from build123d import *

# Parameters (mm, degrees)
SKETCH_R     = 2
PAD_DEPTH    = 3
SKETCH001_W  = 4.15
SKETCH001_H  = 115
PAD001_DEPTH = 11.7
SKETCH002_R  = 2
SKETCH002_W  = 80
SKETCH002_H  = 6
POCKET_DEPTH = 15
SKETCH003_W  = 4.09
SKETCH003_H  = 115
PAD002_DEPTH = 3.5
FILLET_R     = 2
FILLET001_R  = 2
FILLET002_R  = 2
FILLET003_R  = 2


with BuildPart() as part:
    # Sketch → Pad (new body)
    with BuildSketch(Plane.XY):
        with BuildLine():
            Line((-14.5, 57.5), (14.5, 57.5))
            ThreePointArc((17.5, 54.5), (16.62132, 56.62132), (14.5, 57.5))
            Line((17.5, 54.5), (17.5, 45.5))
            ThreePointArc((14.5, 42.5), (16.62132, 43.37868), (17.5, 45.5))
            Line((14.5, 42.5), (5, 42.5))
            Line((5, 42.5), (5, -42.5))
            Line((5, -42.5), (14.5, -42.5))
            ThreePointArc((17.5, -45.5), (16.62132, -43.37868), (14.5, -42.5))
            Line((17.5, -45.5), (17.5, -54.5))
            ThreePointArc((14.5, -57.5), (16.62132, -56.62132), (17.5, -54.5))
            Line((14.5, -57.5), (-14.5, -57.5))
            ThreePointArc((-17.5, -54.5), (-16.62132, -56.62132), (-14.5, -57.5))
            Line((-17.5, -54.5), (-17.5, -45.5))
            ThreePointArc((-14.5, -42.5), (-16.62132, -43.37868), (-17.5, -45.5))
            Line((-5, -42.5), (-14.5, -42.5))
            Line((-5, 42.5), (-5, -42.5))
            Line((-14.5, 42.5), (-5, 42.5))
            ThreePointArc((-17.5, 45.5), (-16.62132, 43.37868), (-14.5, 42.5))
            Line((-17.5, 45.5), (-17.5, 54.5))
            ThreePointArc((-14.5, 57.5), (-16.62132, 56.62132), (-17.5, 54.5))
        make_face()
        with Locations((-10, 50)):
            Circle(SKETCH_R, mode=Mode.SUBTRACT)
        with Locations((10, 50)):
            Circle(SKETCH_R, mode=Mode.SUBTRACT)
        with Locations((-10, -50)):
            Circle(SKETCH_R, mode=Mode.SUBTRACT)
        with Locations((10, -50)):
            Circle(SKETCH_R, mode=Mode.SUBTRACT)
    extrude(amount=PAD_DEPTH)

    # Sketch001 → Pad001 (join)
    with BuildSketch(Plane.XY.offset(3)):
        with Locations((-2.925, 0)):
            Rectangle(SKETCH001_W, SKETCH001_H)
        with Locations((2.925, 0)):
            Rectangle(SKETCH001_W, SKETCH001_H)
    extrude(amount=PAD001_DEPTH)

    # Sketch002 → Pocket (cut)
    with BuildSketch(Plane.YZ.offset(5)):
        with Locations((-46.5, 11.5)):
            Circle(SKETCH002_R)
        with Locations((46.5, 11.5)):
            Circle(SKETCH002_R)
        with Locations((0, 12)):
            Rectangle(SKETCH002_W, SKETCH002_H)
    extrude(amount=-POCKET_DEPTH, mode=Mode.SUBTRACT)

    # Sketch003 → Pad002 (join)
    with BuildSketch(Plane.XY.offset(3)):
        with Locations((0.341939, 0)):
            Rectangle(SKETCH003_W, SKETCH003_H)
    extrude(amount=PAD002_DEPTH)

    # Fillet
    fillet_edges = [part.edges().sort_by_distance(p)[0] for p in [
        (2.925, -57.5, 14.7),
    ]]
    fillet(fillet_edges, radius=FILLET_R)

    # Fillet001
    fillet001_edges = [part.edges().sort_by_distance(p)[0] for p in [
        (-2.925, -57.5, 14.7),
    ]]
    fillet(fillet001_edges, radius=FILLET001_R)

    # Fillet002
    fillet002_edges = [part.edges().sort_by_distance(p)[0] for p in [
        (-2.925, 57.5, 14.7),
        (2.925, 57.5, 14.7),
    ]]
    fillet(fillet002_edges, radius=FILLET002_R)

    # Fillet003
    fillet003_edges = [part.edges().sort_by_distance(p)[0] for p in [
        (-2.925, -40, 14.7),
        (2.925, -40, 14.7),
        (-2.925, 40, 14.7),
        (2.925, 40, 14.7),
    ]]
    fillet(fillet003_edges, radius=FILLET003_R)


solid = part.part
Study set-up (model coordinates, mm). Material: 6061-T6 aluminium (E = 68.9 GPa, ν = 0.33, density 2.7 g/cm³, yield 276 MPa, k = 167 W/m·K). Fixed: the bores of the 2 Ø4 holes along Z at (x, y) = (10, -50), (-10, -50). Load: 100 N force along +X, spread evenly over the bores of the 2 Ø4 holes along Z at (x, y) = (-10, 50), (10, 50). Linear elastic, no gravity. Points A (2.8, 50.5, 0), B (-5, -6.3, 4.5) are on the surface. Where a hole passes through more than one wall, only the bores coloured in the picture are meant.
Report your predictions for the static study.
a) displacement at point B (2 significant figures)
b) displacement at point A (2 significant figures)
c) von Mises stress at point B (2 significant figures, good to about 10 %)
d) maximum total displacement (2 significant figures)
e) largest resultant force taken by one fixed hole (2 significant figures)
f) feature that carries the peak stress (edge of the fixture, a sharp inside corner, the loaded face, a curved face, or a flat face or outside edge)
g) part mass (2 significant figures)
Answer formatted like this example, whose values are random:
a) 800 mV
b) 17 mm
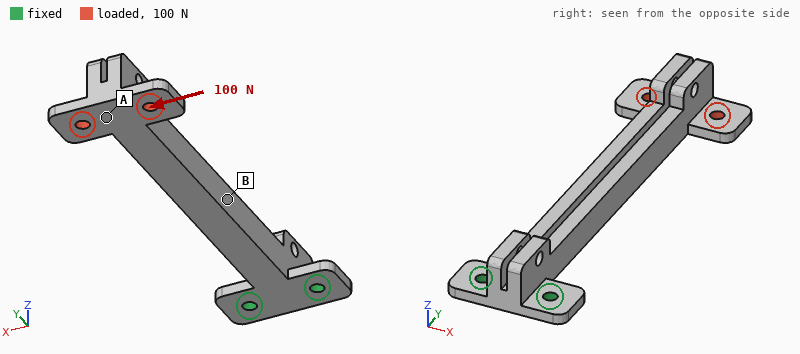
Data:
a) 0.15 mm
b) 0.63 mm
c) 38 MPa
d) 0.70 mm
e) 500 N
f) a flat face or outside edge
g) 36 g
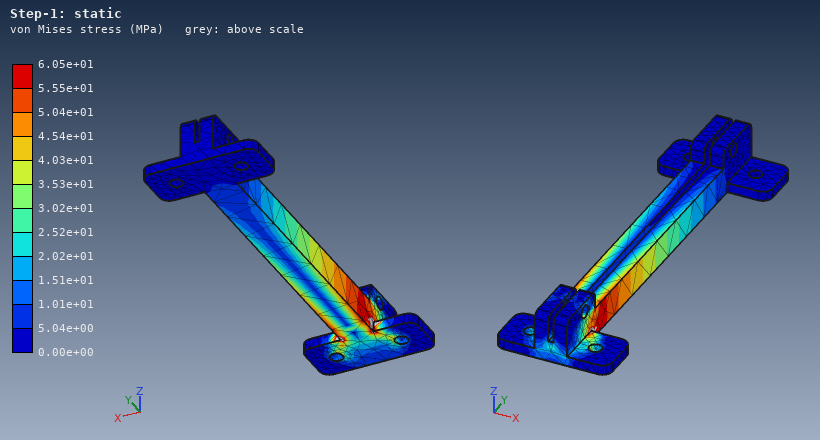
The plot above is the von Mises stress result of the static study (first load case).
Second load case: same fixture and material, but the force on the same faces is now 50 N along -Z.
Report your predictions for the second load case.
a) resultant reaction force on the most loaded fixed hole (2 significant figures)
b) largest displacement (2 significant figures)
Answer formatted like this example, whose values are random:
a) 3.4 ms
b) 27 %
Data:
a) 81 N
b) 0.72 mm
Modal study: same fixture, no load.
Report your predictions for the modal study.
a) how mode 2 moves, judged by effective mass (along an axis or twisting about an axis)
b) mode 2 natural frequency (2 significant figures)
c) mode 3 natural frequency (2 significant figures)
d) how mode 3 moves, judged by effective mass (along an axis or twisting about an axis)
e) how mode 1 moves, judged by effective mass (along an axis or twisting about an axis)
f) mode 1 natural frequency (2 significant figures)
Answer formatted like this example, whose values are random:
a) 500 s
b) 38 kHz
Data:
a) along X
b) 580 Hz
c) 2800 Hz
d) twisting about Y
e) along Z
f) 390 Hz
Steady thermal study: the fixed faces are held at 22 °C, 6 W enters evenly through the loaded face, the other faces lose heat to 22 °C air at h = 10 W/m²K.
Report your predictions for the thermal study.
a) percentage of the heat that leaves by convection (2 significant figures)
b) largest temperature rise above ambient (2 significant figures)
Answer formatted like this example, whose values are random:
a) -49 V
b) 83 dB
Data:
a) 23 %
b) 37 K
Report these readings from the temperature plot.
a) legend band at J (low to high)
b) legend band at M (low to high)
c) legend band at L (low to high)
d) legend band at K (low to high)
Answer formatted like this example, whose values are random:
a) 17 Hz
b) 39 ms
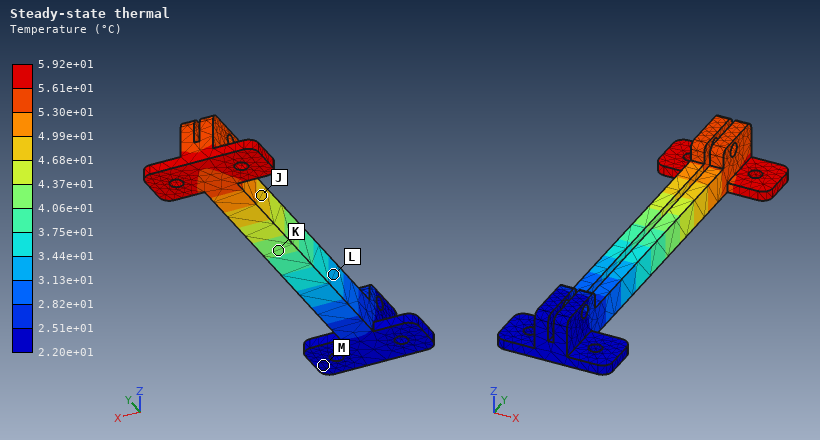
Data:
a) 4.68e+01 to 4.99e+01 °C
b) 2.20e+01 to 2.51e+01 °C
c) 3.13e+01 to 3.44e+01 °C
d) 4.06e+01 to 4.37e+01 °C
